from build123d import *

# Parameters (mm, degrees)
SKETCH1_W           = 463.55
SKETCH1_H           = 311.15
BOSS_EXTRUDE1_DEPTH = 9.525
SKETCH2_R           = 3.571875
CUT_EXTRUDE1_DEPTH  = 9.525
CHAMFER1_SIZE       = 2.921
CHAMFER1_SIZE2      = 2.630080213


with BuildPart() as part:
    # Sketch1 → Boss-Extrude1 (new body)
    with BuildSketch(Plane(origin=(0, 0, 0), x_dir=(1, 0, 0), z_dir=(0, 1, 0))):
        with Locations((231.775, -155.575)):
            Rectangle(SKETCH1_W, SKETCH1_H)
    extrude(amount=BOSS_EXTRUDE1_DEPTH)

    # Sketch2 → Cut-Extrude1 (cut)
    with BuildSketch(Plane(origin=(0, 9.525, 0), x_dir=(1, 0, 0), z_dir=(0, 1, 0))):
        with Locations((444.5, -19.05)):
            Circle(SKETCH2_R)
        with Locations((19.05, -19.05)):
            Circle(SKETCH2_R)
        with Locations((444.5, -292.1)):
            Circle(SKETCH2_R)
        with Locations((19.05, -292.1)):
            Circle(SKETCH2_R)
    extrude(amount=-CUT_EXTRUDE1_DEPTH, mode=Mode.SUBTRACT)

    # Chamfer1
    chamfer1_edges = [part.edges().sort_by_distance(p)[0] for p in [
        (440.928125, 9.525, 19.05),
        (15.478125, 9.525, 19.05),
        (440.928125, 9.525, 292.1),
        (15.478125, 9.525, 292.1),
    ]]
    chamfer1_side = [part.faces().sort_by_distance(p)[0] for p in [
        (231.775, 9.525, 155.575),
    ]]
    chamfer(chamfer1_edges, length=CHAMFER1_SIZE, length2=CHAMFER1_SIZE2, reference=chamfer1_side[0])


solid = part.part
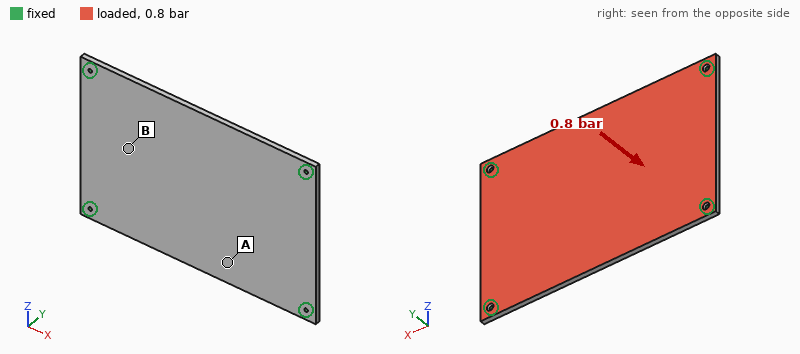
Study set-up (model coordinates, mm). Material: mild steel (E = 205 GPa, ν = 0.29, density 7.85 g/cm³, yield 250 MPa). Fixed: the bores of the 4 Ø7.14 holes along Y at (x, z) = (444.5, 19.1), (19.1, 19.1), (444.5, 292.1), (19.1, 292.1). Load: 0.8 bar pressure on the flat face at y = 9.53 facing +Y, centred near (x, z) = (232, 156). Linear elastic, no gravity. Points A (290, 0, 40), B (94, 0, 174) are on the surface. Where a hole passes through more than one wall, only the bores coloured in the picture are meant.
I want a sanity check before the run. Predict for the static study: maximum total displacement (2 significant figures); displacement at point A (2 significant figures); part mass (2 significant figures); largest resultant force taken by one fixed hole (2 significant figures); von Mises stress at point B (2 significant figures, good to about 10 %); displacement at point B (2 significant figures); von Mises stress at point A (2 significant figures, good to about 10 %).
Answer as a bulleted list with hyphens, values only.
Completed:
- 0.94 mm
- 0.79 mm
- 11 kg
- 3.5 kN
- 26 MPa
- 0.54 mm
- 48 MPa
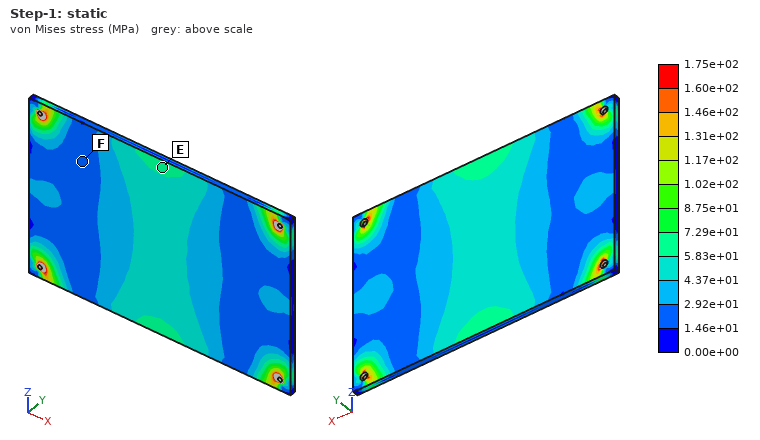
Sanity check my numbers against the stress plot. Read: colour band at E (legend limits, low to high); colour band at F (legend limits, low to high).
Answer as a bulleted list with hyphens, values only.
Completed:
- 5.83e+01 to 7.29e+01 MPa
- 1.46e+01 to 2.92e+01 MPa
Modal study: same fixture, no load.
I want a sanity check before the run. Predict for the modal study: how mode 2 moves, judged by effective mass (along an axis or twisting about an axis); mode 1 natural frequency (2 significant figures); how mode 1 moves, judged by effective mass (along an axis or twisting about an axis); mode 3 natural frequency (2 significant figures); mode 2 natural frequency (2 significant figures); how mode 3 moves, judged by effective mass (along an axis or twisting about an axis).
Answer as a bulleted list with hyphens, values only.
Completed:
- twisting about X
- 200 Hz
- along Y
- 500 Hz
- 340 Hz
- twisting about Z
